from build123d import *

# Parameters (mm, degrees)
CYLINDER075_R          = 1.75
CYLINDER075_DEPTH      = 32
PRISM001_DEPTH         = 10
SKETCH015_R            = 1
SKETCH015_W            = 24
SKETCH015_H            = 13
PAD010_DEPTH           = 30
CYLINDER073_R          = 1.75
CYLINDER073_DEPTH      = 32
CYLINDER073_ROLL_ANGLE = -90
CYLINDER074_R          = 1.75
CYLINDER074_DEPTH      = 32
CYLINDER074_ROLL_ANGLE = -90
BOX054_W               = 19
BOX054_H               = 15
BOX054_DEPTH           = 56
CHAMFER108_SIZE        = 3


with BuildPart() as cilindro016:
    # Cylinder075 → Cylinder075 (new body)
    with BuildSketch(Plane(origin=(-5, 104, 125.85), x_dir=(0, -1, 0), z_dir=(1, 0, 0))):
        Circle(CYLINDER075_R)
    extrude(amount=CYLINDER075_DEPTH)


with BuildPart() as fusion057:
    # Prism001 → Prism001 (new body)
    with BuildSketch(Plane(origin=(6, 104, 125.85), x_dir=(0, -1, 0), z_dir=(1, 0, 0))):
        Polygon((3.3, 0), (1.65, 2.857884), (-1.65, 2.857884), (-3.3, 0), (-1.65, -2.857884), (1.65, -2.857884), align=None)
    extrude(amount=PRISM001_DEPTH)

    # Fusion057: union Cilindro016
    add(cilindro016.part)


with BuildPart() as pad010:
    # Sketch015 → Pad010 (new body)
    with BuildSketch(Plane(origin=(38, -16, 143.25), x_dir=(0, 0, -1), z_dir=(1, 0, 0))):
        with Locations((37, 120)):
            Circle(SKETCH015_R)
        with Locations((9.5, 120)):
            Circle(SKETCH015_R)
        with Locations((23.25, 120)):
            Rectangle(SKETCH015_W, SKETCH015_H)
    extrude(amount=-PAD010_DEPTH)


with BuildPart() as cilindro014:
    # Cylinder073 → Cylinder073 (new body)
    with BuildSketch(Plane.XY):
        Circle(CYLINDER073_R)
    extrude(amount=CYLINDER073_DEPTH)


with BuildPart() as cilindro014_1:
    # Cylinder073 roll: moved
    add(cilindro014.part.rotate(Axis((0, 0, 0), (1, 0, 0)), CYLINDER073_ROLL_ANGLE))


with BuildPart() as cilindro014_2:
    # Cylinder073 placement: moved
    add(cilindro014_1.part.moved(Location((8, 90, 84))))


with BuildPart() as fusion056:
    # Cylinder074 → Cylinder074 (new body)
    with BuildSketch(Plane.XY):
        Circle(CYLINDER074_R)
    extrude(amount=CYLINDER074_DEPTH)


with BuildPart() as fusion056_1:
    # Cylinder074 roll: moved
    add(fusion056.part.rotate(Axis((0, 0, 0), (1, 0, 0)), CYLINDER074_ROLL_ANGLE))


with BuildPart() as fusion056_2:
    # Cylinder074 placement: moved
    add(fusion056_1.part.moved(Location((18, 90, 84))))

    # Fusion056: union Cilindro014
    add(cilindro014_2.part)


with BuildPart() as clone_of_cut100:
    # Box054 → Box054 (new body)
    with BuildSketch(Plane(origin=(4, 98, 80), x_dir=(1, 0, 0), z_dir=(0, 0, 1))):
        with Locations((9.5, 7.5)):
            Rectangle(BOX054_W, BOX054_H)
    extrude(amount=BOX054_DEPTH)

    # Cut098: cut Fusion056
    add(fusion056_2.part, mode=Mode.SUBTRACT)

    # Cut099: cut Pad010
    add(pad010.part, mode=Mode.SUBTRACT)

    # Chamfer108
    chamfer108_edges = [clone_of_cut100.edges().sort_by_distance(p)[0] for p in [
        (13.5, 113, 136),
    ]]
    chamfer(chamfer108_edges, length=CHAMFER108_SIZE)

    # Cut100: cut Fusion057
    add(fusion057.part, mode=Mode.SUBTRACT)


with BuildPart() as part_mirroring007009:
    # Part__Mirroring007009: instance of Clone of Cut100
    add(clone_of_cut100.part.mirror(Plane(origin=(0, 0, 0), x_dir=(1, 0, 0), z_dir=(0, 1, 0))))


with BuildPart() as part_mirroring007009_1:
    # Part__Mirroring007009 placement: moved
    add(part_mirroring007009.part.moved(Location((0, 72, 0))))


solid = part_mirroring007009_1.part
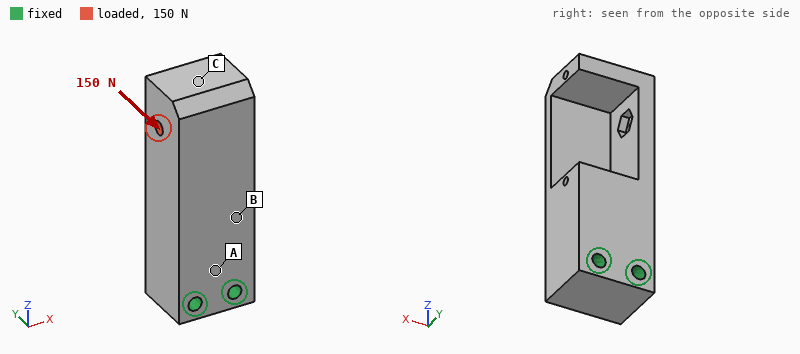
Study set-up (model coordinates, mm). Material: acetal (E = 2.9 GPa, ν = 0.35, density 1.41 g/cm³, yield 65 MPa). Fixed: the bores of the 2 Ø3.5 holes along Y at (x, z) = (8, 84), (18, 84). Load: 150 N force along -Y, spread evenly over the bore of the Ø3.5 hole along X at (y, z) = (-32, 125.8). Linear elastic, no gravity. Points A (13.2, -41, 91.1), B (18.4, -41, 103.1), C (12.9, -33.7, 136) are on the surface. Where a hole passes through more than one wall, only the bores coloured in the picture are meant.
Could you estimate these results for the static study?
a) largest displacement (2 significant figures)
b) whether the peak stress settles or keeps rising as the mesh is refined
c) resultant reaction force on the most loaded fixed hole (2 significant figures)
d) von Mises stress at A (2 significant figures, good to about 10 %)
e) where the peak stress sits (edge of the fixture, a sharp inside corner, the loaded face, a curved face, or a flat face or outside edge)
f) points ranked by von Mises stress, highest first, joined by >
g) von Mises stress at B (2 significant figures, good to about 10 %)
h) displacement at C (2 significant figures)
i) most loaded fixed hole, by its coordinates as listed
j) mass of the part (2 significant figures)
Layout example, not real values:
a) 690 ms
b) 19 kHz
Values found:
a) 0.67 mm
b) keeps rising
c) 120 N
d) 7.3 MPa
e) a sharp inside corner
f) A > B > C
g) 4.1 MPa
h) 0.59 mm
i) (8, 84)
j) 15 g
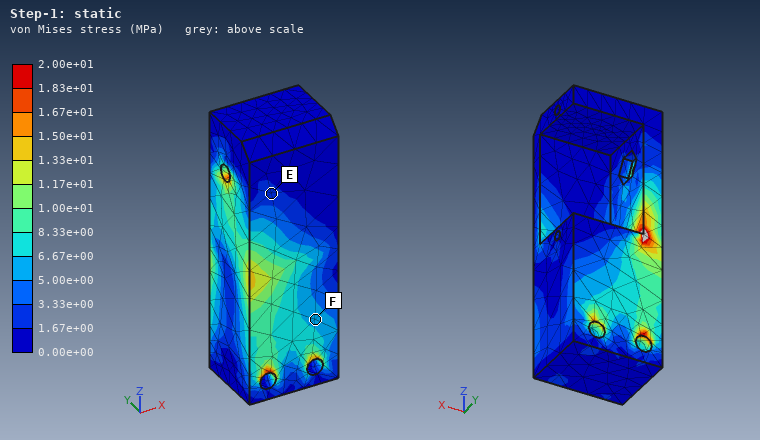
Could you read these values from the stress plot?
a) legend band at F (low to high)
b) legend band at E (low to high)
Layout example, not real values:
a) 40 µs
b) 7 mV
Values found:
a) 5.00e+00 to 6.67e+00 MPa
b) 1.67e+00 to 3.33e+00 MPa
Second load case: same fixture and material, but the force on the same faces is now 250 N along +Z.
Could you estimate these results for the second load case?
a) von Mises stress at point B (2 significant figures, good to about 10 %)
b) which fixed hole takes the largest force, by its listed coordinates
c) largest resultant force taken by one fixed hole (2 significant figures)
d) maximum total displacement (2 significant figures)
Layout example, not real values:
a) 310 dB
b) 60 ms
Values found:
a) 1.2 MPa
b) (8, 84)
c) 290 N
d) 0.22 mm
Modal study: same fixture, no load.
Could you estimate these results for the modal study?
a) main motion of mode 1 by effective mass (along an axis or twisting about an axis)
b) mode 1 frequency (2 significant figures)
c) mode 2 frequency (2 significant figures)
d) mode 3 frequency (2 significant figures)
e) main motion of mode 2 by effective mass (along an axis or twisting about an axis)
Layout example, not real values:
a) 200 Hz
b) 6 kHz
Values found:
a) along Y
b) 1100 Hz
c) 1400 Hz
d) 2600 Hz
e) along X
